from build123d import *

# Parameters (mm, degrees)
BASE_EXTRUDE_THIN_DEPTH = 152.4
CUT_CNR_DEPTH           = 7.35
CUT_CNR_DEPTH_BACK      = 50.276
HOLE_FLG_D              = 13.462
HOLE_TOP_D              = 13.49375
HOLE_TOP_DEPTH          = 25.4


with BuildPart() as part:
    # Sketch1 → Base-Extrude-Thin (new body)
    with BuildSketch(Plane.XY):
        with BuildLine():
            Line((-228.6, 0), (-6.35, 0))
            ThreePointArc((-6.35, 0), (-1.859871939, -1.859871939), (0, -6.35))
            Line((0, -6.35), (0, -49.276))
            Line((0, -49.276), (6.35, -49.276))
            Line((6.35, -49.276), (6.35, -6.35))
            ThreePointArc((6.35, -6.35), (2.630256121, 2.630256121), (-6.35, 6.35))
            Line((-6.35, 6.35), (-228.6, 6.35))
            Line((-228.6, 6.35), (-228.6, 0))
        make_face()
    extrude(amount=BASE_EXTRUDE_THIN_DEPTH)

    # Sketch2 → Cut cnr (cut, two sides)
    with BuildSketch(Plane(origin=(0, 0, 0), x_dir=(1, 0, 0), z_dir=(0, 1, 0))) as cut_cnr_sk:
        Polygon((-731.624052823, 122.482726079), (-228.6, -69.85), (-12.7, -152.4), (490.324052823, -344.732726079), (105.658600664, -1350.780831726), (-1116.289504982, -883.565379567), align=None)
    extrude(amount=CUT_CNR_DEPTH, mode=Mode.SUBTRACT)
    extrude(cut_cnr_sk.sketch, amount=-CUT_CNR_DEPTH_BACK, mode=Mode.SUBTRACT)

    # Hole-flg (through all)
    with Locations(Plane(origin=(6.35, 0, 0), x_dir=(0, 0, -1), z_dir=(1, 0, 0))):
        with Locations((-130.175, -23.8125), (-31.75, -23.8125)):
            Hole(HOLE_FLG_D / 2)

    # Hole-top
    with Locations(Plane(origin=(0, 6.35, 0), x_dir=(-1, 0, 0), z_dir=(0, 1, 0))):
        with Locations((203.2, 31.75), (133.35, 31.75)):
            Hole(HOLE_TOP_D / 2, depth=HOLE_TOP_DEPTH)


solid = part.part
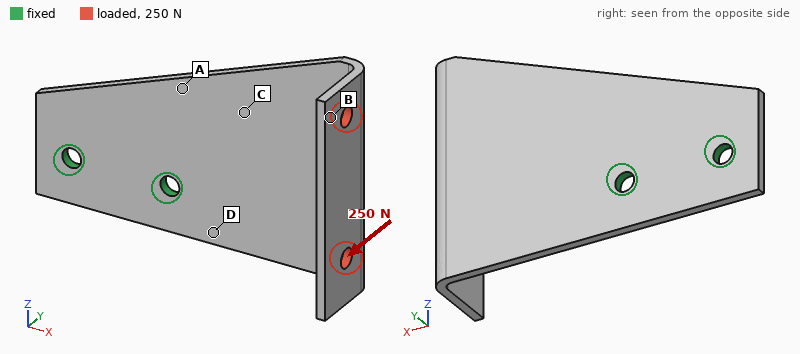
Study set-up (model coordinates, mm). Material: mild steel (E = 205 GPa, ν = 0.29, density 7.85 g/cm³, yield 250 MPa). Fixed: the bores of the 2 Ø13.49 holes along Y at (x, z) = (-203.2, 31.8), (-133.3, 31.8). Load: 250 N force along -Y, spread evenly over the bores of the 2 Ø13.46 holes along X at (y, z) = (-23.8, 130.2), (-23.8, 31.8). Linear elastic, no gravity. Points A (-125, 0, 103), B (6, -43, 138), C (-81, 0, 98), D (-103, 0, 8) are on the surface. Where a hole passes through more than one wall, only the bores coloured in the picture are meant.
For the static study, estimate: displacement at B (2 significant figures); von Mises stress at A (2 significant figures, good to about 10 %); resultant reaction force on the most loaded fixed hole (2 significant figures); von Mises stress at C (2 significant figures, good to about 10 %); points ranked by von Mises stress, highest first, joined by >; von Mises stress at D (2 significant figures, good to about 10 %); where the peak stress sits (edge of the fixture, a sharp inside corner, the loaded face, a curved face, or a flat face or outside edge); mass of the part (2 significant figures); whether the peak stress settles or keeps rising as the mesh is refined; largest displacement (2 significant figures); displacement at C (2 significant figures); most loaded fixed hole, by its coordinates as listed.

0.66 mm
31 MPa
420 N
21 MPa
D > A > C > B
42 MPa
edge of the fixture
1.7 kg
keeps rising
0.70 mm
0.17 mm
(-133.3, 31.8)
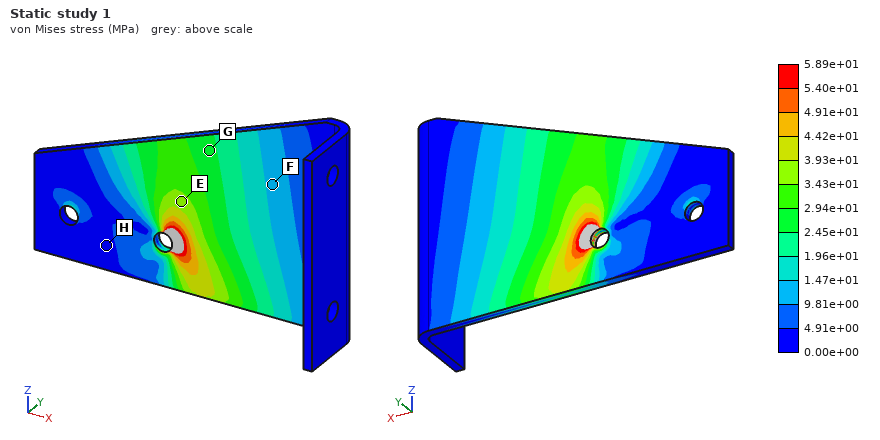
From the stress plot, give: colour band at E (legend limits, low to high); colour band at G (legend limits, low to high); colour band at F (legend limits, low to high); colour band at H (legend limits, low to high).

3.43e+01 to 3.93e+01 MPa
2.45e+01 to 2.94e+01 MPa
9.81e+00 to 1.47e+01 MPa
0.00e+00 to 4.91e+00 MPa
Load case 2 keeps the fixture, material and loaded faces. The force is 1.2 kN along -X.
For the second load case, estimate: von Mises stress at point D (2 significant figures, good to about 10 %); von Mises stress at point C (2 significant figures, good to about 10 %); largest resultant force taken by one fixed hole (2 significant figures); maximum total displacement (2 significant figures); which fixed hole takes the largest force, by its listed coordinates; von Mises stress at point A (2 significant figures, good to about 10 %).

46 MPa
38 MPa
1.0 kN
0.84 mm
(-133.3, 31.8)
37 MPa
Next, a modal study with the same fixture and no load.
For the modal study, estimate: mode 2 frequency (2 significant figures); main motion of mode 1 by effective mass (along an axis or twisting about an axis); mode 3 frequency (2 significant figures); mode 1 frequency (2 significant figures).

310 Hz
along Y
740 Hz
140 Hz
